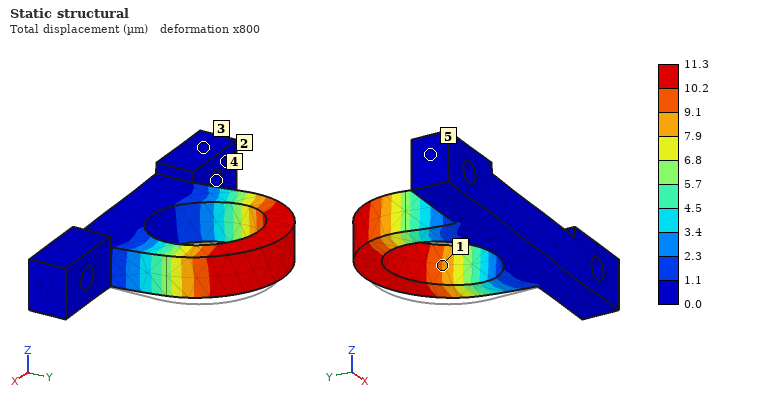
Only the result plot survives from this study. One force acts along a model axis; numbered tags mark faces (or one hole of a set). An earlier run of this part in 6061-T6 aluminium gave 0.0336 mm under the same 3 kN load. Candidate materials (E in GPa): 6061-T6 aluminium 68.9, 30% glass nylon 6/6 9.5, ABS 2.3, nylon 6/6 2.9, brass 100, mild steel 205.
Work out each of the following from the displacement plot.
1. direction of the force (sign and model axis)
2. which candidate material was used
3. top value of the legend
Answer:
-X
mild steel
11.3 µm
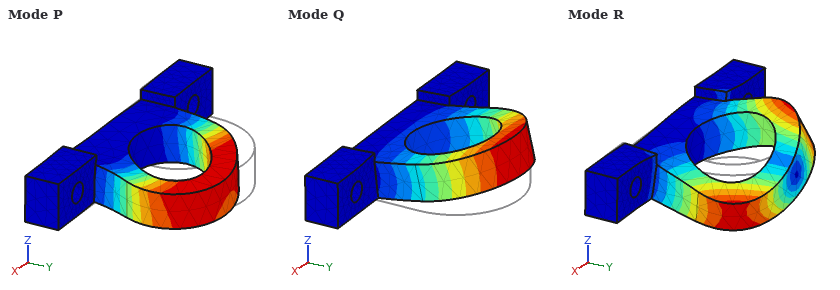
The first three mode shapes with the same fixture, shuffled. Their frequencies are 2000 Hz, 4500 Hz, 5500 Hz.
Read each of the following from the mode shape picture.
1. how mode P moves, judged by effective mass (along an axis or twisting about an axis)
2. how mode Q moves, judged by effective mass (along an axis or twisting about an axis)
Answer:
along X
along Z
